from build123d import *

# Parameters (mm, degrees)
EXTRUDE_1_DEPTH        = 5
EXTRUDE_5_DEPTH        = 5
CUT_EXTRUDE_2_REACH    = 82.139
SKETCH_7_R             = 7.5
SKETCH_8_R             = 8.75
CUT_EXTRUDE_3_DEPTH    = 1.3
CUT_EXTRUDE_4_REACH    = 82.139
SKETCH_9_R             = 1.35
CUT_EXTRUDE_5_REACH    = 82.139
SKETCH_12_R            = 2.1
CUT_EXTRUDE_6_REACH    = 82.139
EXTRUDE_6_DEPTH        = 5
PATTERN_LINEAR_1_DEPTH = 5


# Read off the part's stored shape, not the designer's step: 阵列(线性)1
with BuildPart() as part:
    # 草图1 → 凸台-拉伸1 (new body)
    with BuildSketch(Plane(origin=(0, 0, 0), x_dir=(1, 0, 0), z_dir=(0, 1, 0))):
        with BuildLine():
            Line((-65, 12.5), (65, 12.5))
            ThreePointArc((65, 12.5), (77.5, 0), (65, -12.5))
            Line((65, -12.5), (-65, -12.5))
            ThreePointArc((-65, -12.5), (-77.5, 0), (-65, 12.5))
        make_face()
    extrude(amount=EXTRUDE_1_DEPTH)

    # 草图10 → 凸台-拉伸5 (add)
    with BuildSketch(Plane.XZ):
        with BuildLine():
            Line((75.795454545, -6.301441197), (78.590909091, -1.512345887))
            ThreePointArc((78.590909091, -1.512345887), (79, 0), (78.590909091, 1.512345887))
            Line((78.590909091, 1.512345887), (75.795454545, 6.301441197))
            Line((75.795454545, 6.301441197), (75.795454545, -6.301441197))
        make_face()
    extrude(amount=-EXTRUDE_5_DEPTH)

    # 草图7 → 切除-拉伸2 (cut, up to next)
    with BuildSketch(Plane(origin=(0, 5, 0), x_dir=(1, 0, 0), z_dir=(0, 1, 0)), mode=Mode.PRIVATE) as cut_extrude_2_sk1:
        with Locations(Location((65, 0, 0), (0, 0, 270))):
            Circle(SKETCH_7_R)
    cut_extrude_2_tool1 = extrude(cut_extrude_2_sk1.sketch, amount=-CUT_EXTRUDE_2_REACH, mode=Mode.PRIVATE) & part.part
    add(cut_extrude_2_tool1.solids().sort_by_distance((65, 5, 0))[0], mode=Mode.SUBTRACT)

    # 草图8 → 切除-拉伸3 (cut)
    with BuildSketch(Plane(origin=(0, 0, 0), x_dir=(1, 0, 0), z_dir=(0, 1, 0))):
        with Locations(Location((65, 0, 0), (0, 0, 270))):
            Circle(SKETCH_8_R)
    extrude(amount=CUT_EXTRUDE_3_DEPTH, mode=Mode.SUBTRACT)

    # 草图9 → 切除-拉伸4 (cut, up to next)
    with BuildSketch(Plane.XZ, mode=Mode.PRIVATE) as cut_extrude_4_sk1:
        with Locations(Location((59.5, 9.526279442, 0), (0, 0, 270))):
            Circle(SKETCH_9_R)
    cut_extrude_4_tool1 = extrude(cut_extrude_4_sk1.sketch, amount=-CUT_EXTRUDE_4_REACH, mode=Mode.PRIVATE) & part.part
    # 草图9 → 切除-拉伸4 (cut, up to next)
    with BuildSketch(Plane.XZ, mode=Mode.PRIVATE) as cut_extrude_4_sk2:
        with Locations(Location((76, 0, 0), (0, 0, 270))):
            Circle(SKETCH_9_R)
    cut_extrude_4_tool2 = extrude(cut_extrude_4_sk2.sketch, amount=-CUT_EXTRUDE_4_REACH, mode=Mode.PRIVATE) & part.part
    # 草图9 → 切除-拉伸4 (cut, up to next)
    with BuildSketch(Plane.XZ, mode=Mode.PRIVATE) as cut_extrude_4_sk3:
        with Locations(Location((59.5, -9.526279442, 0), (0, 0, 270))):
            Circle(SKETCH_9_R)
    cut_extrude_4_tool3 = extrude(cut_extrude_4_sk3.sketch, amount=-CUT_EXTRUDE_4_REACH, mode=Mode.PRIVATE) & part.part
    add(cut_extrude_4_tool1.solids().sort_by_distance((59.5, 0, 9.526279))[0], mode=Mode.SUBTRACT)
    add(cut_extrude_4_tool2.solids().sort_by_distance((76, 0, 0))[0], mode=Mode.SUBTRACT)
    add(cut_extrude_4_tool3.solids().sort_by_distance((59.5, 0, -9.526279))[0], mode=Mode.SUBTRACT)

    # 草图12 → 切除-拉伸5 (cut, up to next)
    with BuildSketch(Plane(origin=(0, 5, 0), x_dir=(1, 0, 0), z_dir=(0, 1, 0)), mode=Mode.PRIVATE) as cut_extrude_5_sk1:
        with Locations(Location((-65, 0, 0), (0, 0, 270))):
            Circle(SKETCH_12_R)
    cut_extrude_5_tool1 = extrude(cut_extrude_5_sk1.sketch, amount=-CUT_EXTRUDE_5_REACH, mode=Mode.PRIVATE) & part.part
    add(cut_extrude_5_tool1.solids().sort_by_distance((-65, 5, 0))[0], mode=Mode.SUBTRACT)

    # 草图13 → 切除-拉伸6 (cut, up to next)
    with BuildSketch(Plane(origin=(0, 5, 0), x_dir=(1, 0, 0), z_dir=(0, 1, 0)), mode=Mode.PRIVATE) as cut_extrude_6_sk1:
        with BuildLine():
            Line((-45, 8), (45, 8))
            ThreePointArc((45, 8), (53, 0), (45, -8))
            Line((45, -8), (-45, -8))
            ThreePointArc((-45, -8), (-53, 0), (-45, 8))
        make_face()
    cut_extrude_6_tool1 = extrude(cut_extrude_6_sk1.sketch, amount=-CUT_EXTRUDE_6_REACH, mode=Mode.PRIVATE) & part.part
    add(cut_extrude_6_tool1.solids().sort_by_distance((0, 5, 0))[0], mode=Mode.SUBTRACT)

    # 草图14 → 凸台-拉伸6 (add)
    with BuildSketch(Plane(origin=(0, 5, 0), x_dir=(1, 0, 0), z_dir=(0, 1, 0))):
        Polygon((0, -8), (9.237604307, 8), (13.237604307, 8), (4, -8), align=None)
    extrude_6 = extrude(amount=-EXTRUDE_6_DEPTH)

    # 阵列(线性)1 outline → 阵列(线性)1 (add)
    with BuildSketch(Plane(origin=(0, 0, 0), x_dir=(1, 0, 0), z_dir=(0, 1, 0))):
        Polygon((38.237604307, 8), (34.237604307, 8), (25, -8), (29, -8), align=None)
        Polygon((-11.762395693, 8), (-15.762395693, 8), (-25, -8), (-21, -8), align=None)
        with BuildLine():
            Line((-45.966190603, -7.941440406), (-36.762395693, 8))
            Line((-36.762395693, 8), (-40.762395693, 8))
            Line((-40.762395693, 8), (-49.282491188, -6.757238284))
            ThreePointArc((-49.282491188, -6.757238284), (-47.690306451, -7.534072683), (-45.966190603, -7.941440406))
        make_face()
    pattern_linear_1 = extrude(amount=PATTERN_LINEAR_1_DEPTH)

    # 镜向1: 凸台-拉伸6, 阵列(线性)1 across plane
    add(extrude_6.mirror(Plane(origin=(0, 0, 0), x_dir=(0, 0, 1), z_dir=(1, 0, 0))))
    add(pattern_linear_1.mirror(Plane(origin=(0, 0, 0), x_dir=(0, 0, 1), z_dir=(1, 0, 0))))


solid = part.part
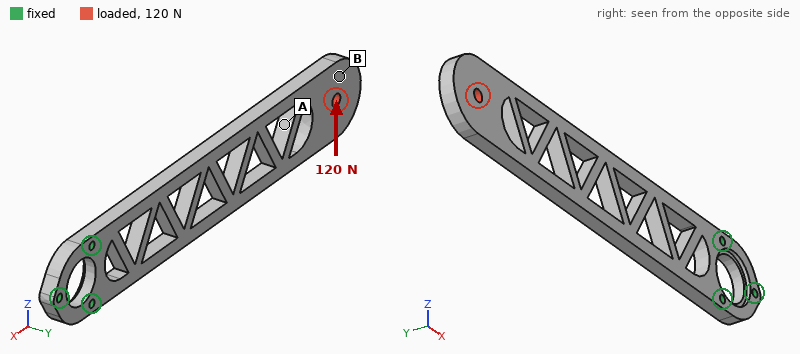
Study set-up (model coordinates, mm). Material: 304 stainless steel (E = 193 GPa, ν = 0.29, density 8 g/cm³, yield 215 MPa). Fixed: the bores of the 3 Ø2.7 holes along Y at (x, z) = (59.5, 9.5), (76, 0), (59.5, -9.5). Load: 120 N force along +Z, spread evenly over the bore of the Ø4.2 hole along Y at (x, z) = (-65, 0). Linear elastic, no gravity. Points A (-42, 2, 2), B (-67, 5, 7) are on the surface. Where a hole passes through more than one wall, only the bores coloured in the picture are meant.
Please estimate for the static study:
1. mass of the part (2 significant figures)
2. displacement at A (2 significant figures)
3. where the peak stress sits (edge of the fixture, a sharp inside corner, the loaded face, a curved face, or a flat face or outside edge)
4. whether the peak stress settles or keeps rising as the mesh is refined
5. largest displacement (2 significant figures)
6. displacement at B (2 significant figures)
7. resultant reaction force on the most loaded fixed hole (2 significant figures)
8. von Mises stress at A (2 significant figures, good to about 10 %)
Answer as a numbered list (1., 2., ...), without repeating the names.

1. 96 g
2. 0.067 mm
3. edge of the fixture
4. keeps rising
5. 0.10 mm
6. 0.091 mm
7. 740 N
8. 6.7 MPa
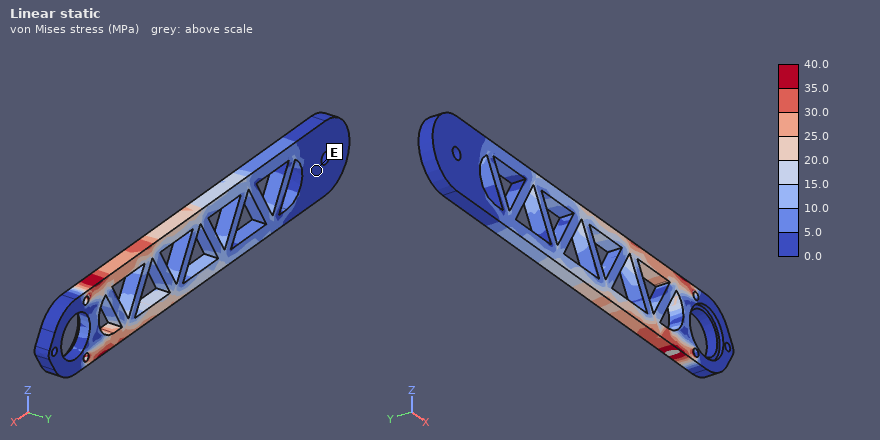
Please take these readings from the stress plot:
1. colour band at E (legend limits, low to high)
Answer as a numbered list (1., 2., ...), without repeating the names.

1. 0.0 to 5.0 MPa
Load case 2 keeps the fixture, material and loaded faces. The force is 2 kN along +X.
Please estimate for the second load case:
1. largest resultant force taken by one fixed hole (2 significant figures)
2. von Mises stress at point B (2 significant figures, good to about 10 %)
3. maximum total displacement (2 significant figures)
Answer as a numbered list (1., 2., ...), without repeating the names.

1. 1000 N
2. 13 MPa
3. 27 µm
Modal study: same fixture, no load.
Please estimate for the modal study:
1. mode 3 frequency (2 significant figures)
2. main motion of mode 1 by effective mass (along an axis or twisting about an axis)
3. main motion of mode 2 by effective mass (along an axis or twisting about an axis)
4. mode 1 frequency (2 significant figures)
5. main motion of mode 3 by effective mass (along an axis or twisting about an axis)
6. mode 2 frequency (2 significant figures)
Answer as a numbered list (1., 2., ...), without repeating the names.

1. 1100 Hz
2. along Y
3. along Z
4. 170 Hz
5. along Y
6. 1000 Hz
